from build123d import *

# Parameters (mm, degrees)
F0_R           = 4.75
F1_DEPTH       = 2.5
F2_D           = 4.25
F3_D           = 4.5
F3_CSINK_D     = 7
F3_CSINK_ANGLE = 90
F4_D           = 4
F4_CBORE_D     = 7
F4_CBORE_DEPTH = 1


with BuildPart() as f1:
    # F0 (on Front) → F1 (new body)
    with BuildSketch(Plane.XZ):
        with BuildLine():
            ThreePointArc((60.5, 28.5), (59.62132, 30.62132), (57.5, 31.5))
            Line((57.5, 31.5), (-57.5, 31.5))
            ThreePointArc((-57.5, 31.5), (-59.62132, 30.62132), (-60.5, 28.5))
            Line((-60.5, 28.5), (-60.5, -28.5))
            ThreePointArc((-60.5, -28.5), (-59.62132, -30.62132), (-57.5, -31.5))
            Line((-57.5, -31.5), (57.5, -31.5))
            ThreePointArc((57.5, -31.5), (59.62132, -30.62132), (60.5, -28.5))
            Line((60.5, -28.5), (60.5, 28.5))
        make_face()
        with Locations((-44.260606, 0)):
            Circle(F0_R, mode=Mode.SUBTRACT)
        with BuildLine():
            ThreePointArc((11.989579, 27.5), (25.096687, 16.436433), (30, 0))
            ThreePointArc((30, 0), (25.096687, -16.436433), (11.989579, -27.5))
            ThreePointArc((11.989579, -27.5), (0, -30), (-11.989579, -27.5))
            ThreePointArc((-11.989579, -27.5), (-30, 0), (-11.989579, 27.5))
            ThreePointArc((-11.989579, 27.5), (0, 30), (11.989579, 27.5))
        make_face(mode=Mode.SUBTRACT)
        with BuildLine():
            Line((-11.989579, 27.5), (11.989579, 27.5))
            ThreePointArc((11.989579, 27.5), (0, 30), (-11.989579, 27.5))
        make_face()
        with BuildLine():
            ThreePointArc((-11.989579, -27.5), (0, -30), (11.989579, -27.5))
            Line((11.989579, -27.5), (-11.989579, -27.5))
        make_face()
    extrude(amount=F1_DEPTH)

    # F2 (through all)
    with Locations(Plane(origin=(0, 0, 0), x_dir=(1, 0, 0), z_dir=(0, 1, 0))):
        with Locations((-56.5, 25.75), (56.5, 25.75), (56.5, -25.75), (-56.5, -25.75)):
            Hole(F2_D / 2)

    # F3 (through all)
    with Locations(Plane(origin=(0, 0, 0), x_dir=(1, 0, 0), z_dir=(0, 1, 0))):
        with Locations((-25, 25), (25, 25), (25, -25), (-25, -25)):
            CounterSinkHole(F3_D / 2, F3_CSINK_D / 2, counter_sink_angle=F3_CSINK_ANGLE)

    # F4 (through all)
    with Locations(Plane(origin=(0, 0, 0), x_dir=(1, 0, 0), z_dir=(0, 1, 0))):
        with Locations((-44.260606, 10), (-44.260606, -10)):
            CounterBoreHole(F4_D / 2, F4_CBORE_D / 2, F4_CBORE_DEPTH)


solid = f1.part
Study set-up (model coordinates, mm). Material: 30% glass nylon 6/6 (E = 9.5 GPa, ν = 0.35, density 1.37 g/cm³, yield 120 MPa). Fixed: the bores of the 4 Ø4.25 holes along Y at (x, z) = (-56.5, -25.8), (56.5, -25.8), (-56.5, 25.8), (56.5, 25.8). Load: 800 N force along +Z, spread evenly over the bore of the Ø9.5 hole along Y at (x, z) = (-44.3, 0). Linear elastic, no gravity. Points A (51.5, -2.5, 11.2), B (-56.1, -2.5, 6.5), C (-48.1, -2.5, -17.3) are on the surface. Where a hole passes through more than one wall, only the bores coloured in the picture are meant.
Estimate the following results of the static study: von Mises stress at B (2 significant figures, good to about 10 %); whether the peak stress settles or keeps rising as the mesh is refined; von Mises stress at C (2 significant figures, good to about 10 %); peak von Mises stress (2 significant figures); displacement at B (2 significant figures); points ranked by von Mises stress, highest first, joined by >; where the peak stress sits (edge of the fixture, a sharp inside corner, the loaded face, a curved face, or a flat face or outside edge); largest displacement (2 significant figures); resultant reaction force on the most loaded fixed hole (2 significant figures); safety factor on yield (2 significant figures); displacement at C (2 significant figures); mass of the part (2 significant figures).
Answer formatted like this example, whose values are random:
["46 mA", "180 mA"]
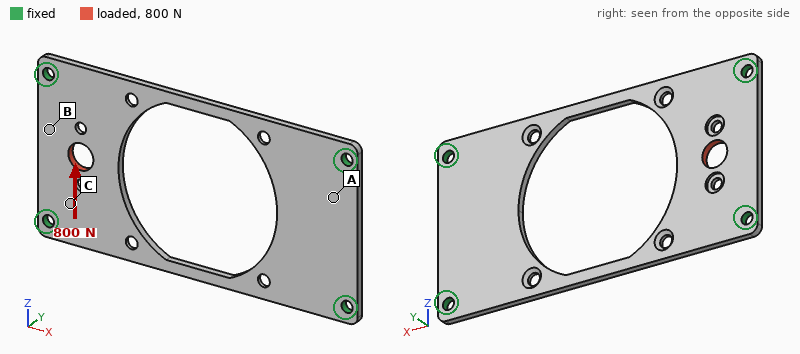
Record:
["5.6 MPa", "settles", "8.5 MPa", "52 MPa", "19 µm", "C > B > A", "a curved face", "55 µm", "430 N", "2.3", "22 µm", "16 g"]
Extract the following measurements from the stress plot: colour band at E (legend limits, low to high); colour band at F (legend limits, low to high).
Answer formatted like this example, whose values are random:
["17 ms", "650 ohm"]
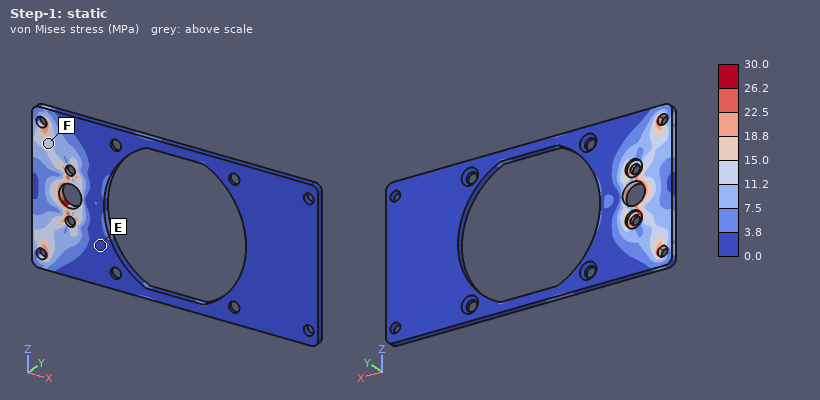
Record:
["0.0 to 3.8 MPa", "11.2 to 15.0 MPa"]
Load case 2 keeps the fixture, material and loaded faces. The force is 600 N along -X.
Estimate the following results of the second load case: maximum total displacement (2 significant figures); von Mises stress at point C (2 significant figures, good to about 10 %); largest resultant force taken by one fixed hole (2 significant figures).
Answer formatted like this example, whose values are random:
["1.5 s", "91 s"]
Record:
["58 µm", "9.8 MPa", "340 N"]
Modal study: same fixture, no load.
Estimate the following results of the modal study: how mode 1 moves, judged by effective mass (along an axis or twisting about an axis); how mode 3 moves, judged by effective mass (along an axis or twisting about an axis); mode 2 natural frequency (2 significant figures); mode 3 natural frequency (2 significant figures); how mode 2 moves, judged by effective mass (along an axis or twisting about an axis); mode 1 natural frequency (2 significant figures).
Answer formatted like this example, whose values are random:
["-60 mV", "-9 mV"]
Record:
["along Y", "twisting about Z", "920 Hz", "1200 Hz", "twisting about X", "700 Hz"]
